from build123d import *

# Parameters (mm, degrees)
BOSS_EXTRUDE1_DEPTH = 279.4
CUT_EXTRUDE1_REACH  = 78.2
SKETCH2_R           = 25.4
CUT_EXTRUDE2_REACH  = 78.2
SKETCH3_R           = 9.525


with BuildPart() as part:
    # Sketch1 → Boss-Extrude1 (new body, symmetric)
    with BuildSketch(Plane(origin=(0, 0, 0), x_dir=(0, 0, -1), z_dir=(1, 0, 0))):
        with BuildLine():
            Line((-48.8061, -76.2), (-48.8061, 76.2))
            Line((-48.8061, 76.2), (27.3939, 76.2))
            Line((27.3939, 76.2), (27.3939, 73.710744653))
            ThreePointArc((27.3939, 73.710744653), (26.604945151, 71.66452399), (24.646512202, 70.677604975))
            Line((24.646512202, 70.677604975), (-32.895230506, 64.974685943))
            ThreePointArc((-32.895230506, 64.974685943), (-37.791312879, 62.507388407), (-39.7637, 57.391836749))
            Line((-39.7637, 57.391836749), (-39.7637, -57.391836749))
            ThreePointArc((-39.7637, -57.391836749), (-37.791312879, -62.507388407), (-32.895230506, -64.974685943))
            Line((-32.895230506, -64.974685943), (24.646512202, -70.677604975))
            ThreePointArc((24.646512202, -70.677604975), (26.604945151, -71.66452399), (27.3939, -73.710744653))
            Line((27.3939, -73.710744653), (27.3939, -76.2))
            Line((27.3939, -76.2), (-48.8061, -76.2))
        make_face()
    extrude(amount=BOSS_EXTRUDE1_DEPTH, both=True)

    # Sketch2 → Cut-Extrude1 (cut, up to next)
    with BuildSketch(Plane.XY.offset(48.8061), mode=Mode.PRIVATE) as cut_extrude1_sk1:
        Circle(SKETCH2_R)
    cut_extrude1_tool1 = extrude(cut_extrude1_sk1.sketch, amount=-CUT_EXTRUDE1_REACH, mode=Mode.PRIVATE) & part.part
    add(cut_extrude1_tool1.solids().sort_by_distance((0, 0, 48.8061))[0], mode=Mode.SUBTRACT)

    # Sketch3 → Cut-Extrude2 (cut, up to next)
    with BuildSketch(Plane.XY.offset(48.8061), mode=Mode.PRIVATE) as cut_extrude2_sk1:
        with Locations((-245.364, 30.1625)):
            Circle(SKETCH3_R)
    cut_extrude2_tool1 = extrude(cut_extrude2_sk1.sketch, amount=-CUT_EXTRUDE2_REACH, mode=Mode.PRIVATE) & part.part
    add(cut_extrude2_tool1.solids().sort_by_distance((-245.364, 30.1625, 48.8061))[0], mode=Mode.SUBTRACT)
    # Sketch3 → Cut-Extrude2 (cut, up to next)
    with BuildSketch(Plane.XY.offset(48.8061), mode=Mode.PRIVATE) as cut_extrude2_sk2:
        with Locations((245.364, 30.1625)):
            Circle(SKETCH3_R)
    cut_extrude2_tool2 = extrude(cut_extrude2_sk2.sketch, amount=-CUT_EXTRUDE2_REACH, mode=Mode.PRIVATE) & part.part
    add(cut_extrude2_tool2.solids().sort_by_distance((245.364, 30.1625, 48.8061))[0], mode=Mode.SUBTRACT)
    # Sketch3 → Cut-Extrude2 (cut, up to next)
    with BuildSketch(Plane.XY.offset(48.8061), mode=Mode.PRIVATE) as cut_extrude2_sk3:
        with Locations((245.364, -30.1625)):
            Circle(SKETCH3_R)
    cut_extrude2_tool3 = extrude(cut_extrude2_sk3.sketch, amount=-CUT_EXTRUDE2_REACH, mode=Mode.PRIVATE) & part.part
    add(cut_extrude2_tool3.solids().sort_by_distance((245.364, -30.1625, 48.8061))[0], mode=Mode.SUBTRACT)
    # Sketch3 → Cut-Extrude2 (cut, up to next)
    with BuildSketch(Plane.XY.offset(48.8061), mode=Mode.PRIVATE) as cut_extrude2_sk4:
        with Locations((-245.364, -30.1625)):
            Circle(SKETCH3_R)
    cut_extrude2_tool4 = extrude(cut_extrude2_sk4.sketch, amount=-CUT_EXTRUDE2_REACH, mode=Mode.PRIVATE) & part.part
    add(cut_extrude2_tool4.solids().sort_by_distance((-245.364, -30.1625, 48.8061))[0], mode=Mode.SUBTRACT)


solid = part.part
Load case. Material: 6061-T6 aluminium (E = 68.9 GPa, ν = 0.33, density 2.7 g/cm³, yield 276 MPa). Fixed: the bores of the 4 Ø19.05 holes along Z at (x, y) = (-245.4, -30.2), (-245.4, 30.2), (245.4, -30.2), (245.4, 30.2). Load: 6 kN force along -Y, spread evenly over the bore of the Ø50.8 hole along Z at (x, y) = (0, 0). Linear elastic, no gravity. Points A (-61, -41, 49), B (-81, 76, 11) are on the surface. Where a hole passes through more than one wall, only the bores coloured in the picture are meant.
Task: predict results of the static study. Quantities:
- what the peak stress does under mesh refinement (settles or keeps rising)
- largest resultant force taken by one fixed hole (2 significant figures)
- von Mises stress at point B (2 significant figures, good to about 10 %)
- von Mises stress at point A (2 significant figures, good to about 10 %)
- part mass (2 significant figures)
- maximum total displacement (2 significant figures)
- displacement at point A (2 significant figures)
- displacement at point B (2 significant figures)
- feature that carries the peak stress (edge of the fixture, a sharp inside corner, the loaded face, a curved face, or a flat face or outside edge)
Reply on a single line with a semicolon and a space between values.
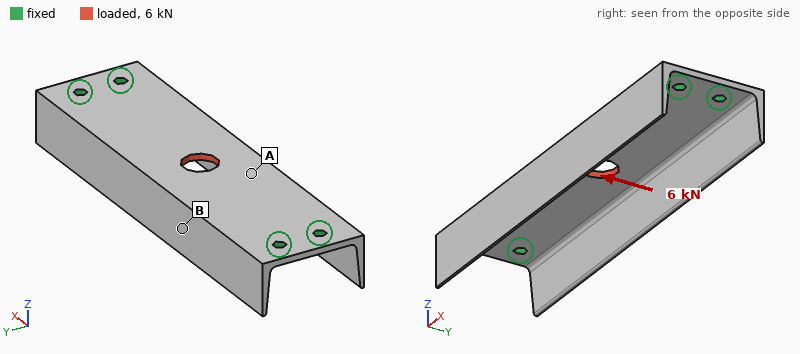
keeps rising; 3.5 kN; 1.9 MPa; 4.3 MPa; 3.8 kg; 85 µm; 40 µm; 57 µm; edge of the fixture
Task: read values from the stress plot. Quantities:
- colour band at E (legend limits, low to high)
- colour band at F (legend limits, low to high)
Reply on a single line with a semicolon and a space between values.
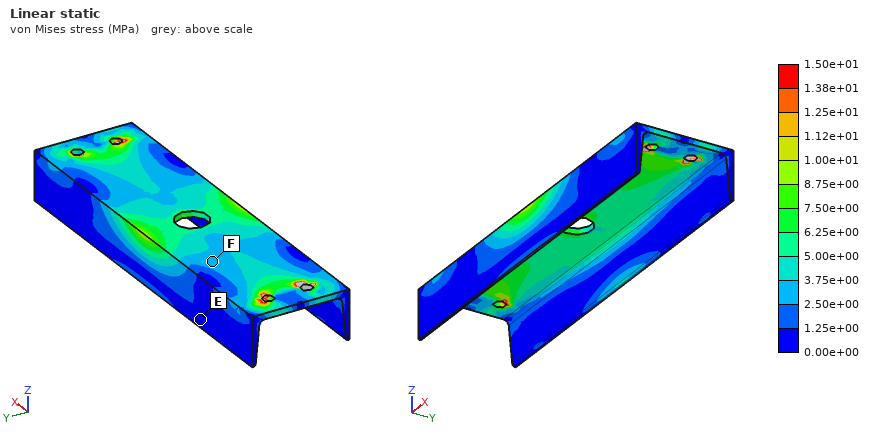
0.00e+00 to 1.25e+00 MPa; 2.50e+00 to 3.75e+00 MPa
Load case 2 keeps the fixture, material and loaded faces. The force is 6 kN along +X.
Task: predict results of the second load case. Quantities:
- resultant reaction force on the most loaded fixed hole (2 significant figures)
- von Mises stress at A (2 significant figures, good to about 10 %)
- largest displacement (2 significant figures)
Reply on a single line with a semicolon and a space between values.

1.5 kN; 2.4 MPa; 8.7 µm
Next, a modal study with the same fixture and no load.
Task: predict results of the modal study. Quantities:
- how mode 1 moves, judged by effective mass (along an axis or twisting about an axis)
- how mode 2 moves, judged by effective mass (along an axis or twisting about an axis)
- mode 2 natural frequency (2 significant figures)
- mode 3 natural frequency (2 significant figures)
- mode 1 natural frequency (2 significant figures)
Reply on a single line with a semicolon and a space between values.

along Y; along Z; 640 Hz; 800 Hz; 560 Hz
